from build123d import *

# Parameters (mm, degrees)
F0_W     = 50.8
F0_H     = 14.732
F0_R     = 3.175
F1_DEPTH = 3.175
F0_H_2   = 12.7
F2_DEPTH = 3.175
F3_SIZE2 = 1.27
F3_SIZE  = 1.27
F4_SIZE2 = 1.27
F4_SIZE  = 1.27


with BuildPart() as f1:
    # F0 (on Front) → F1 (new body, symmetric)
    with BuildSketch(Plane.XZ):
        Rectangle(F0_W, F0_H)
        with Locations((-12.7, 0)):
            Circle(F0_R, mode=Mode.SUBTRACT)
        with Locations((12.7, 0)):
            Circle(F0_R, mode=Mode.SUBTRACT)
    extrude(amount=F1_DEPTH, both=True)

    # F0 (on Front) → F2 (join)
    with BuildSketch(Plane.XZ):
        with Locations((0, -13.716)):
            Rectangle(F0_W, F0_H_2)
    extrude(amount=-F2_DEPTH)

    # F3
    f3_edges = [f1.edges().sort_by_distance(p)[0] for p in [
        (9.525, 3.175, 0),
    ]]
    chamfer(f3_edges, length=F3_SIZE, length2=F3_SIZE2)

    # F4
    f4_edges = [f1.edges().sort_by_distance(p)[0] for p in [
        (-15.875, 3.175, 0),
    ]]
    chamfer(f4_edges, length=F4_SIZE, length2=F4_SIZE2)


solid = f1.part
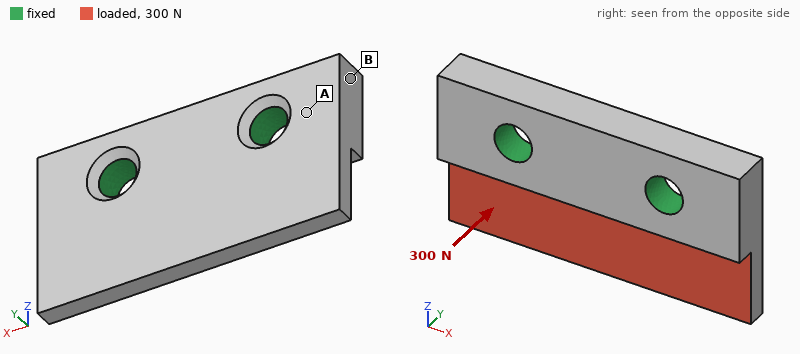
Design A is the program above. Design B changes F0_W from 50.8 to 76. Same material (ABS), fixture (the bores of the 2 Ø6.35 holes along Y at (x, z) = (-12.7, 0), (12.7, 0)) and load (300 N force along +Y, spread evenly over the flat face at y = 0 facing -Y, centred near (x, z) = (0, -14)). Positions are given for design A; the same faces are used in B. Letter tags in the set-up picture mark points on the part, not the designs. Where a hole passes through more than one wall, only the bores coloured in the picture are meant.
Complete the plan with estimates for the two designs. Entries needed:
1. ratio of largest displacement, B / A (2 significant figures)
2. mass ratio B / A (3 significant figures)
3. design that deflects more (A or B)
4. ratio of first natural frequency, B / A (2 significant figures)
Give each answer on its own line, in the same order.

1.4
1.53
B
0.63
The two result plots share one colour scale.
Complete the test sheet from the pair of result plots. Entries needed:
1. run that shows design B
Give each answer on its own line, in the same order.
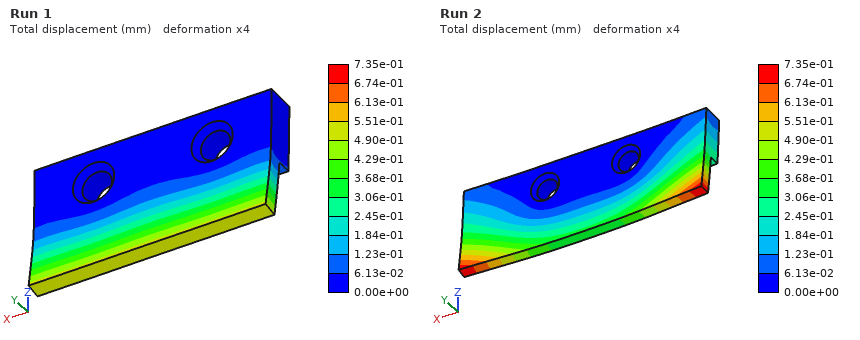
Run 2
